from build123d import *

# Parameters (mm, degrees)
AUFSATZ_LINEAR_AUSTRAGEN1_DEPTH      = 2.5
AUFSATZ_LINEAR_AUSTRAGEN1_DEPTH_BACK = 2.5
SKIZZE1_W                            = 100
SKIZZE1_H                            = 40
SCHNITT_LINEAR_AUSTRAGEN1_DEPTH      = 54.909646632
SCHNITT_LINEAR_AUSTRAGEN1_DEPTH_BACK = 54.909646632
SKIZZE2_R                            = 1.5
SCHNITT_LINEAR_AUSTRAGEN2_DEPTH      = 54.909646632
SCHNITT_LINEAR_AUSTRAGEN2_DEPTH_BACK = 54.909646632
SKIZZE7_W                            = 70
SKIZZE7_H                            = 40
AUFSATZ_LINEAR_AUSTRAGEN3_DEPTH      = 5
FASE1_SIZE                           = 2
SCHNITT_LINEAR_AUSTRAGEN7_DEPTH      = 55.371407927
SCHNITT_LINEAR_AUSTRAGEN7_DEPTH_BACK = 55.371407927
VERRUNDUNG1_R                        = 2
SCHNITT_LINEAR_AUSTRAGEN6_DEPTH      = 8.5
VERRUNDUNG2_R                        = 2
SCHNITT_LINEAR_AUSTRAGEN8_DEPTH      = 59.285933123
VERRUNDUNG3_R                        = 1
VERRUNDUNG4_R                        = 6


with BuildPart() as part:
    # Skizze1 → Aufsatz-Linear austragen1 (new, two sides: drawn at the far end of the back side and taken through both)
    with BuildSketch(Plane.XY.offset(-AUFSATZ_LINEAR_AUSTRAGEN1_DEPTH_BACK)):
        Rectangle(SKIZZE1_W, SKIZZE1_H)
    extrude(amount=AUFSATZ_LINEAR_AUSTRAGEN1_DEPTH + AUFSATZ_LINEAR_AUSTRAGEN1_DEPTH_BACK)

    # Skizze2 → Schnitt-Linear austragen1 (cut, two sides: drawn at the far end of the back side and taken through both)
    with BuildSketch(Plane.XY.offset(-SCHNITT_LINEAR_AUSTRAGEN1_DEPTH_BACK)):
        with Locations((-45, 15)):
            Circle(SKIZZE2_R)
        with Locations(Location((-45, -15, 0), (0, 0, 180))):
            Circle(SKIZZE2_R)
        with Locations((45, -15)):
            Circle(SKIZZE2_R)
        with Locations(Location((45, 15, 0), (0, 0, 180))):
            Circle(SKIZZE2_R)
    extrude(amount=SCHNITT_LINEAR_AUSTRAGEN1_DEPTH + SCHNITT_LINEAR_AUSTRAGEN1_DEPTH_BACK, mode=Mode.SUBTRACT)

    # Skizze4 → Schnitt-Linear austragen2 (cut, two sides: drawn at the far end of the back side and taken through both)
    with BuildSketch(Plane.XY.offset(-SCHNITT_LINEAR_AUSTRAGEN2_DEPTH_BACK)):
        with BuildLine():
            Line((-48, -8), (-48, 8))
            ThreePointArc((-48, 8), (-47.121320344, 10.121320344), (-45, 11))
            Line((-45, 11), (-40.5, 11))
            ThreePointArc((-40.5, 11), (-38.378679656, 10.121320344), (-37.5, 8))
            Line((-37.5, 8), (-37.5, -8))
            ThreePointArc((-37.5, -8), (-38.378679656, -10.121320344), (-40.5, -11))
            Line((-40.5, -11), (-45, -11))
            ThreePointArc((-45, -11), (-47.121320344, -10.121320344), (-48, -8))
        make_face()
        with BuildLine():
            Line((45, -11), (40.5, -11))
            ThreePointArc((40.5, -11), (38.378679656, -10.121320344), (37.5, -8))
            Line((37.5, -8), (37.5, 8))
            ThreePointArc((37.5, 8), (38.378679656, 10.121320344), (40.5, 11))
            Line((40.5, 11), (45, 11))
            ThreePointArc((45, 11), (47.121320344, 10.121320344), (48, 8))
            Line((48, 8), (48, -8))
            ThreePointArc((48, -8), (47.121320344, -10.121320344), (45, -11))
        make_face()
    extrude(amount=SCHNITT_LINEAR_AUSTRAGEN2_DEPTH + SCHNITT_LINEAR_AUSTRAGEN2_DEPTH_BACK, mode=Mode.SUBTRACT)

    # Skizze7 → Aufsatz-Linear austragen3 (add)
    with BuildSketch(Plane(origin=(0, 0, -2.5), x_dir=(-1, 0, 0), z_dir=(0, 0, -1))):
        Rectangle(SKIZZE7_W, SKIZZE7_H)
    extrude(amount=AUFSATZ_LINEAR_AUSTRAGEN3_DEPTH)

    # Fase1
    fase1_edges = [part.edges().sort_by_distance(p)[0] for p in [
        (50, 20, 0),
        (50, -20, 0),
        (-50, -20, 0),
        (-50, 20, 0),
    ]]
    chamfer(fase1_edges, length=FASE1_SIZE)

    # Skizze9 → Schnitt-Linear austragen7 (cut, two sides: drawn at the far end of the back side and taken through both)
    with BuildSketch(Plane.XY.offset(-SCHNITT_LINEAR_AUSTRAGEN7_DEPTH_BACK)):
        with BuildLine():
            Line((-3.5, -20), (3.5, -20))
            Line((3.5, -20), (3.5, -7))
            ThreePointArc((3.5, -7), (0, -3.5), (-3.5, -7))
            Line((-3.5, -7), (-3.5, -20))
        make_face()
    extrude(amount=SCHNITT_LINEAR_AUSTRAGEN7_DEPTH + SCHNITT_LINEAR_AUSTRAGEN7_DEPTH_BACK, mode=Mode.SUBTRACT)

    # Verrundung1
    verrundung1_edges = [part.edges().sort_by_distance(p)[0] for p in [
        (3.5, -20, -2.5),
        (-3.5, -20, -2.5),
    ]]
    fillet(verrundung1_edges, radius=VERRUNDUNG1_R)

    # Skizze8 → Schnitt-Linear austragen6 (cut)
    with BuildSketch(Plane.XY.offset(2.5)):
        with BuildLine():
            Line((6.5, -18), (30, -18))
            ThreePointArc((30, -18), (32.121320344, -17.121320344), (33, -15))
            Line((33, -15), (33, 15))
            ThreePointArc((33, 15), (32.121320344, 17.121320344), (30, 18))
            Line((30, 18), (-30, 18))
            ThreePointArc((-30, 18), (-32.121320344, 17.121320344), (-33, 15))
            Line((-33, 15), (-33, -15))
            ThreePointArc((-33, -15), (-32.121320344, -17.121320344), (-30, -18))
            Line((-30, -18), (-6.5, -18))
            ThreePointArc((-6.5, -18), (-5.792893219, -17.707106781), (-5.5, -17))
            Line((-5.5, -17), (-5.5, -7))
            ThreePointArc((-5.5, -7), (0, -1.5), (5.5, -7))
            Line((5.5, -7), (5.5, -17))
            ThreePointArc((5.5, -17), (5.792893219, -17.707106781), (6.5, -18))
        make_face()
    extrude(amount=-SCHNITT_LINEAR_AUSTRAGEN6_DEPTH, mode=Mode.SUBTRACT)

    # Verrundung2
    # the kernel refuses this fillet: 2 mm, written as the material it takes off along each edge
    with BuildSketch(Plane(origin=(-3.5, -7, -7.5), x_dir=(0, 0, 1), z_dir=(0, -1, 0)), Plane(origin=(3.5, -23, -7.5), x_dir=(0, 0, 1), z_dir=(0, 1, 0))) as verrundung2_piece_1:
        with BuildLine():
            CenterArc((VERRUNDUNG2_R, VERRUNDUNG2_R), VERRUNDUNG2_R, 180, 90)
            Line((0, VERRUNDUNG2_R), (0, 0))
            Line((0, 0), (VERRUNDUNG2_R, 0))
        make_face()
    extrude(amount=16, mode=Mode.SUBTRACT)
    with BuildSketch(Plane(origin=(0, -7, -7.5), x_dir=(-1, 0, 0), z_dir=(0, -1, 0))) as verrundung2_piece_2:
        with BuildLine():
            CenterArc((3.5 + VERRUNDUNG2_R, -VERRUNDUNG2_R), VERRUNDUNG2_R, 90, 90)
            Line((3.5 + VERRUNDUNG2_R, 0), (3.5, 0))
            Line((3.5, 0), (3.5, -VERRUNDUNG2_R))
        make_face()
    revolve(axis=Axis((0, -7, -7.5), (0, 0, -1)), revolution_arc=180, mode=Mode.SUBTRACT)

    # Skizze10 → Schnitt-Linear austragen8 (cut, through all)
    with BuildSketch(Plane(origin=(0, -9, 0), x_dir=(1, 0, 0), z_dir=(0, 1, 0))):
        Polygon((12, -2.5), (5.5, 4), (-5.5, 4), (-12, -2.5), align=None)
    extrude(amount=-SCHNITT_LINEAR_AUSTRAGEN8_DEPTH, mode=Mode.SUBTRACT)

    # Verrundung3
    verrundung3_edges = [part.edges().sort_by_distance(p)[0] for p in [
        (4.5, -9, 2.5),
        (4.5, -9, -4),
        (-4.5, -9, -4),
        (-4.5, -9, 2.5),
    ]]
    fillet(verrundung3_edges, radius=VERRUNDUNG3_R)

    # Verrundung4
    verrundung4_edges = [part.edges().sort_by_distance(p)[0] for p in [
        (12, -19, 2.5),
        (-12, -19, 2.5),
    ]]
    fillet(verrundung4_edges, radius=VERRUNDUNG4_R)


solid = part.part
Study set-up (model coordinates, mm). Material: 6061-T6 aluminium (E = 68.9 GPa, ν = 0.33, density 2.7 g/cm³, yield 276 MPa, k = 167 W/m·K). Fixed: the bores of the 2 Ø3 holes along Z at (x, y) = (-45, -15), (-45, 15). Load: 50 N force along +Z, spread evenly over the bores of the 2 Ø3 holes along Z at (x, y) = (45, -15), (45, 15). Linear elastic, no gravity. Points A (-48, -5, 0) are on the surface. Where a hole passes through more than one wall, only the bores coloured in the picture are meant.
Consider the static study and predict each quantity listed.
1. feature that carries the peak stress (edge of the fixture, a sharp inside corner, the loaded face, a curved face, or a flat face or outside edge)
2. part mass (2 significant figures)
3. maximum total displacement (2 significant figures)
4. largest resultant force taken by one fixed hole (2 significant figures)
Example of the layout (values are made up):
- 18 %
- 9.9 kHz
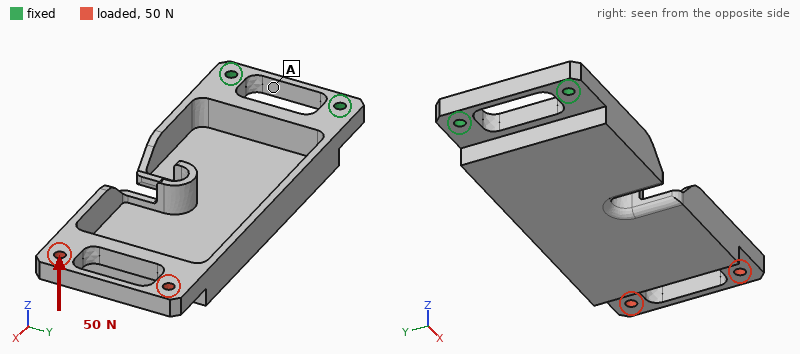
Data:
- a curved face
- 31 g
- 1.1 mm
- 90 N
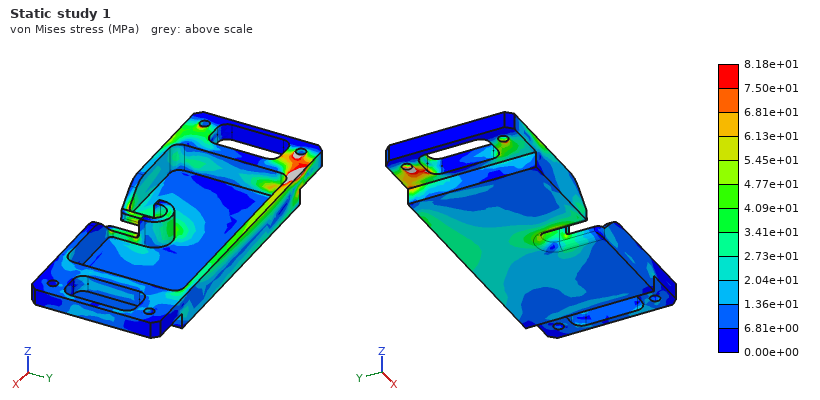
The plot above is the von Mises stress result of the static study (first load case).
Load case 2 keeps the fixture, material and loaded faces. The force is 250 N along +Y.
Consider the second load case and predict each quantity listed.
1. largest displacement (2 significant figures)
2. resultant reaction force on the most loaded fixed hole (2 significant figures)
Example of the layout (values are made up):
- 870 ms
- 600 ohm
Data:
- 1.1 mm
- 660 N
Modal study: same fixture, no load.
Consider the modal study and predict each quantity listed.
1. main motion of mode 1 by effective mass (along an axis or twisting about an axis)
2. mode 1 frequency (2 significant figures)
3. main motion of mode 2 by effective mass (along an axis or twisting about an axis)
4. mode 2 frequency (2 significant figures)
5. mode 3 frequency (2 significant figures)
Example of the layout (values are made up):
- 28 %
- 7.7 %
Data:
- along Z
- 390 Hz
- along Y
- 790 Hz
- 1700 Hz
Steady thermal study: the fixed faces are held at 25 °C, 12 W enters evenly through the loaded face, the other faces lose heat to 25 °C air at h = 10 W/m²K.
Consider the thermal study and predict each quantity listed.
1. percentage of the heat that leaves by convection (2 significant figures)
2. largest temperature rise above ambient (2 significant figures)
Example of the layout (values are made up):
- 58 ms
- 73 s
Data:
- 30 %
- 68 K
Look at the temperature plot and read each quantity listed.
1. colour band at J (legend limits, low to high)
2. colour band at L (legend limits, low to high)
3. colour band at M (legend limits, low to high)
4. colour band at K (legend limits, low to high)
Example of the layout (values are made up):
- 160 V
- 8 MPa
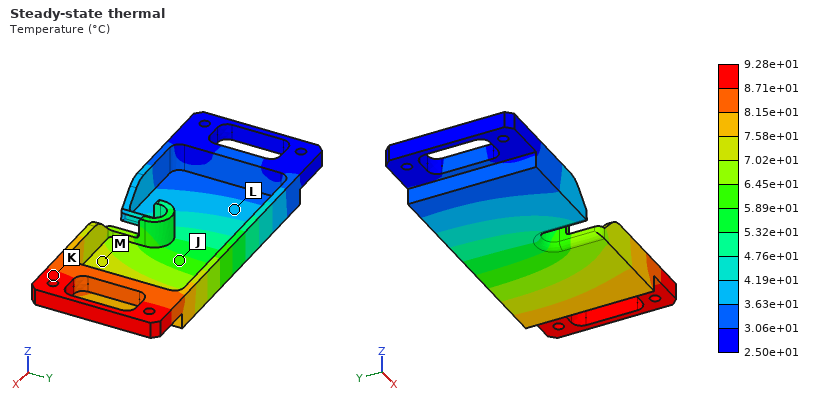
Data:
- 5.89e+01 to 6.45e+01 °C
- 3.63e+01 to 4.19e+01 °C
- 7.02e+01 to 7.58e+01 °C
- 8.71e+01 to 9.28e+01 °C
